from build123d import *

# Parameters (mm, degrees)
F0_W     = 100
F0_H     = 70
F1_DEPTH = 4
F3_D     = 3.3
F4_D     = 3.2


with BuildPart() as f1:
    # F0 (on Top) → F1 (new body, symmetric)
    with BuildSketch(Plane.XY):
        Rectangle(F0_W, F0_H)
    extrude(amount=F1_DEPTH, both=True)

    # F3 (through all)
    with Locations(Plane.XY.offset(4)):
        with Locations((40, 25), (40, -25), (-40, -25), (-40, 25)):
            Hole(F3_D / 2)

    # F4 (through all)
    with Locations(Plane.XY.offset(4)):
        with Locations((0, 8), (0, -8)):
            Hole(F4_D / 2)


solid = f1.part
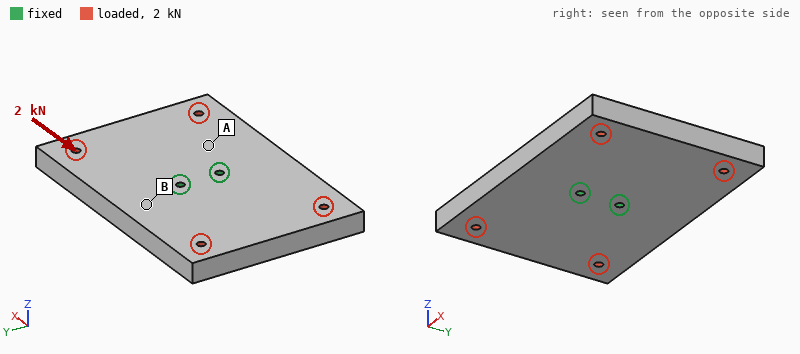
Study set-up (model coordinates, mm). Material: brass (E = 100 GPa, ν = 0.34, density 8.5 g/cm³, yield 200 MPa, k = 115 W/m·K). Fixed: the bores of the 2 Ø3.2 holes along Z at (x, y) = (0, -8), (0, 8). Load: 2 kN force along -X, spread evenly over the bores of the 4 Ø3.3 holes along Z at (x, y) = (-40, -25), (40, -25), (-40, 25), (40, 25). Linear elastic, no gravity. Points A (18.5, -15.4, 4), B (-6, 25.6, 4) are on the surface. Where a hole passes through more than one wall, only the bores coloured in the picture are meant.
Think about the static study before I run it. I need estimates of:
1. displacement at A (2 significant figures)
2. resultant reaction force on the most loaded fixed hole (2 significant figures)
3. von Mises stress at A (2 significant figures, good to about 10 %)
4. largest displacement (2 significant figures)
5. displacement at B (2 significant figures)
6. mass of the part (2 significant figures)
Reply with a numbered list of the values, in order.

1. 1.0 µm
2. 1.0 kN
3. 3.0 MPa
4. 2.1 µm
5. 1.2 µm
6. 470 g
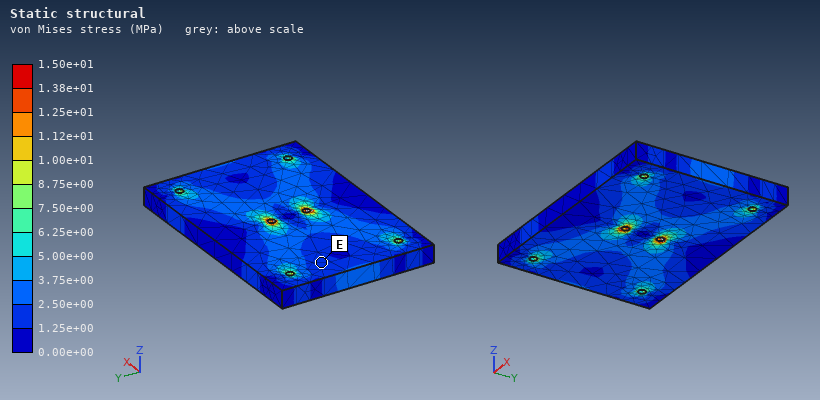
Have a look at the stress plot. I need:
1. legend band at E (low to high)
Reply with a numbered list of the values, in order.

1. 1.25e+00 to 2.50e+00 MPa
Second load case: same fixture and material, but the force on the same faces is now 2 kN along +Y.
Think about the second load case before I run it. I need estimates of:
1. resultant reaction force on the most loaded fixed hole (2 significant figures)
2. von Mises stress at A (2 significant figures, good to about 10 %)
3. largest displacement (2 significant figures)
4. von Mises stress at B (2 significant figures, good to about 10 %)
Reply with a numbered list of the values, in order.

1. 1.0 kN
2. 3.8 MPa
3. 4.5 µm
4. 4.3 MPa
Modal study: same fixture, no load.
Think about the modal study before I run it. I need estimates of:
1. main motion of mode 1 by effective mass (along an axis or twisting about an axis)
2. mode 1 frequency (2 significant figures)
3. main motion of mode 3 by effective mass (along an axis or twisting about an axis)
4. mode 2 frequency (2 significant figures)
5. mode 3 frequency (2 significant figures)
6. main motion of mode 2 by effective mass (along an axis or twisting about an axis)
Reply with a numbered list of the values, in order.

1. twisting about Y
2. 1200 Hz
3. twisting about X
4. 1800 Hz
5. 2400 Hz
6. along Z
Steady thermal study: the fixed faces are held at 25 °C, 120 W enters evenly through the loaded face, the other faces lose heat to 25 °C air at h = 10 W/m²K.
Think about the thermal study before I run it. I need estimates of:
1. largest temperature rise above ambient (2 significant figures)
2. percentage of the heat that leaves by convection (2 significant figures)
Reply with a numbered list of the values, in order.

1. 63 K
2. 5.5 %
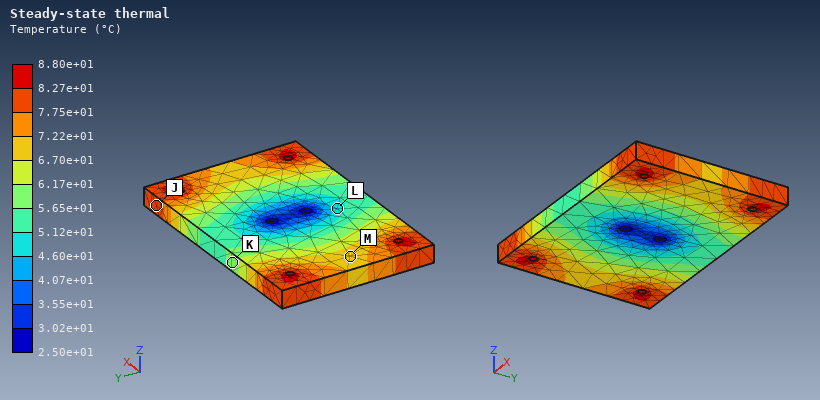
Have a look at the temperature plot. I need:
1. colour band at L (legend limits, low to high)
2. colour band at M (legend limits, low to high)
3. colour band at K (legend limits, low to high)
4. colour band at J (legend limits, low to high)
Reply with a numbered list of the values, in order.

1. 4.60e+01 to 5.12e+01 °C
2. 6.70e+01 to 7.22e+01 °C
3. 5.65e+01 to 6.17e+01 °C
4. 7.75e+01 to 8.27e+01 °C
